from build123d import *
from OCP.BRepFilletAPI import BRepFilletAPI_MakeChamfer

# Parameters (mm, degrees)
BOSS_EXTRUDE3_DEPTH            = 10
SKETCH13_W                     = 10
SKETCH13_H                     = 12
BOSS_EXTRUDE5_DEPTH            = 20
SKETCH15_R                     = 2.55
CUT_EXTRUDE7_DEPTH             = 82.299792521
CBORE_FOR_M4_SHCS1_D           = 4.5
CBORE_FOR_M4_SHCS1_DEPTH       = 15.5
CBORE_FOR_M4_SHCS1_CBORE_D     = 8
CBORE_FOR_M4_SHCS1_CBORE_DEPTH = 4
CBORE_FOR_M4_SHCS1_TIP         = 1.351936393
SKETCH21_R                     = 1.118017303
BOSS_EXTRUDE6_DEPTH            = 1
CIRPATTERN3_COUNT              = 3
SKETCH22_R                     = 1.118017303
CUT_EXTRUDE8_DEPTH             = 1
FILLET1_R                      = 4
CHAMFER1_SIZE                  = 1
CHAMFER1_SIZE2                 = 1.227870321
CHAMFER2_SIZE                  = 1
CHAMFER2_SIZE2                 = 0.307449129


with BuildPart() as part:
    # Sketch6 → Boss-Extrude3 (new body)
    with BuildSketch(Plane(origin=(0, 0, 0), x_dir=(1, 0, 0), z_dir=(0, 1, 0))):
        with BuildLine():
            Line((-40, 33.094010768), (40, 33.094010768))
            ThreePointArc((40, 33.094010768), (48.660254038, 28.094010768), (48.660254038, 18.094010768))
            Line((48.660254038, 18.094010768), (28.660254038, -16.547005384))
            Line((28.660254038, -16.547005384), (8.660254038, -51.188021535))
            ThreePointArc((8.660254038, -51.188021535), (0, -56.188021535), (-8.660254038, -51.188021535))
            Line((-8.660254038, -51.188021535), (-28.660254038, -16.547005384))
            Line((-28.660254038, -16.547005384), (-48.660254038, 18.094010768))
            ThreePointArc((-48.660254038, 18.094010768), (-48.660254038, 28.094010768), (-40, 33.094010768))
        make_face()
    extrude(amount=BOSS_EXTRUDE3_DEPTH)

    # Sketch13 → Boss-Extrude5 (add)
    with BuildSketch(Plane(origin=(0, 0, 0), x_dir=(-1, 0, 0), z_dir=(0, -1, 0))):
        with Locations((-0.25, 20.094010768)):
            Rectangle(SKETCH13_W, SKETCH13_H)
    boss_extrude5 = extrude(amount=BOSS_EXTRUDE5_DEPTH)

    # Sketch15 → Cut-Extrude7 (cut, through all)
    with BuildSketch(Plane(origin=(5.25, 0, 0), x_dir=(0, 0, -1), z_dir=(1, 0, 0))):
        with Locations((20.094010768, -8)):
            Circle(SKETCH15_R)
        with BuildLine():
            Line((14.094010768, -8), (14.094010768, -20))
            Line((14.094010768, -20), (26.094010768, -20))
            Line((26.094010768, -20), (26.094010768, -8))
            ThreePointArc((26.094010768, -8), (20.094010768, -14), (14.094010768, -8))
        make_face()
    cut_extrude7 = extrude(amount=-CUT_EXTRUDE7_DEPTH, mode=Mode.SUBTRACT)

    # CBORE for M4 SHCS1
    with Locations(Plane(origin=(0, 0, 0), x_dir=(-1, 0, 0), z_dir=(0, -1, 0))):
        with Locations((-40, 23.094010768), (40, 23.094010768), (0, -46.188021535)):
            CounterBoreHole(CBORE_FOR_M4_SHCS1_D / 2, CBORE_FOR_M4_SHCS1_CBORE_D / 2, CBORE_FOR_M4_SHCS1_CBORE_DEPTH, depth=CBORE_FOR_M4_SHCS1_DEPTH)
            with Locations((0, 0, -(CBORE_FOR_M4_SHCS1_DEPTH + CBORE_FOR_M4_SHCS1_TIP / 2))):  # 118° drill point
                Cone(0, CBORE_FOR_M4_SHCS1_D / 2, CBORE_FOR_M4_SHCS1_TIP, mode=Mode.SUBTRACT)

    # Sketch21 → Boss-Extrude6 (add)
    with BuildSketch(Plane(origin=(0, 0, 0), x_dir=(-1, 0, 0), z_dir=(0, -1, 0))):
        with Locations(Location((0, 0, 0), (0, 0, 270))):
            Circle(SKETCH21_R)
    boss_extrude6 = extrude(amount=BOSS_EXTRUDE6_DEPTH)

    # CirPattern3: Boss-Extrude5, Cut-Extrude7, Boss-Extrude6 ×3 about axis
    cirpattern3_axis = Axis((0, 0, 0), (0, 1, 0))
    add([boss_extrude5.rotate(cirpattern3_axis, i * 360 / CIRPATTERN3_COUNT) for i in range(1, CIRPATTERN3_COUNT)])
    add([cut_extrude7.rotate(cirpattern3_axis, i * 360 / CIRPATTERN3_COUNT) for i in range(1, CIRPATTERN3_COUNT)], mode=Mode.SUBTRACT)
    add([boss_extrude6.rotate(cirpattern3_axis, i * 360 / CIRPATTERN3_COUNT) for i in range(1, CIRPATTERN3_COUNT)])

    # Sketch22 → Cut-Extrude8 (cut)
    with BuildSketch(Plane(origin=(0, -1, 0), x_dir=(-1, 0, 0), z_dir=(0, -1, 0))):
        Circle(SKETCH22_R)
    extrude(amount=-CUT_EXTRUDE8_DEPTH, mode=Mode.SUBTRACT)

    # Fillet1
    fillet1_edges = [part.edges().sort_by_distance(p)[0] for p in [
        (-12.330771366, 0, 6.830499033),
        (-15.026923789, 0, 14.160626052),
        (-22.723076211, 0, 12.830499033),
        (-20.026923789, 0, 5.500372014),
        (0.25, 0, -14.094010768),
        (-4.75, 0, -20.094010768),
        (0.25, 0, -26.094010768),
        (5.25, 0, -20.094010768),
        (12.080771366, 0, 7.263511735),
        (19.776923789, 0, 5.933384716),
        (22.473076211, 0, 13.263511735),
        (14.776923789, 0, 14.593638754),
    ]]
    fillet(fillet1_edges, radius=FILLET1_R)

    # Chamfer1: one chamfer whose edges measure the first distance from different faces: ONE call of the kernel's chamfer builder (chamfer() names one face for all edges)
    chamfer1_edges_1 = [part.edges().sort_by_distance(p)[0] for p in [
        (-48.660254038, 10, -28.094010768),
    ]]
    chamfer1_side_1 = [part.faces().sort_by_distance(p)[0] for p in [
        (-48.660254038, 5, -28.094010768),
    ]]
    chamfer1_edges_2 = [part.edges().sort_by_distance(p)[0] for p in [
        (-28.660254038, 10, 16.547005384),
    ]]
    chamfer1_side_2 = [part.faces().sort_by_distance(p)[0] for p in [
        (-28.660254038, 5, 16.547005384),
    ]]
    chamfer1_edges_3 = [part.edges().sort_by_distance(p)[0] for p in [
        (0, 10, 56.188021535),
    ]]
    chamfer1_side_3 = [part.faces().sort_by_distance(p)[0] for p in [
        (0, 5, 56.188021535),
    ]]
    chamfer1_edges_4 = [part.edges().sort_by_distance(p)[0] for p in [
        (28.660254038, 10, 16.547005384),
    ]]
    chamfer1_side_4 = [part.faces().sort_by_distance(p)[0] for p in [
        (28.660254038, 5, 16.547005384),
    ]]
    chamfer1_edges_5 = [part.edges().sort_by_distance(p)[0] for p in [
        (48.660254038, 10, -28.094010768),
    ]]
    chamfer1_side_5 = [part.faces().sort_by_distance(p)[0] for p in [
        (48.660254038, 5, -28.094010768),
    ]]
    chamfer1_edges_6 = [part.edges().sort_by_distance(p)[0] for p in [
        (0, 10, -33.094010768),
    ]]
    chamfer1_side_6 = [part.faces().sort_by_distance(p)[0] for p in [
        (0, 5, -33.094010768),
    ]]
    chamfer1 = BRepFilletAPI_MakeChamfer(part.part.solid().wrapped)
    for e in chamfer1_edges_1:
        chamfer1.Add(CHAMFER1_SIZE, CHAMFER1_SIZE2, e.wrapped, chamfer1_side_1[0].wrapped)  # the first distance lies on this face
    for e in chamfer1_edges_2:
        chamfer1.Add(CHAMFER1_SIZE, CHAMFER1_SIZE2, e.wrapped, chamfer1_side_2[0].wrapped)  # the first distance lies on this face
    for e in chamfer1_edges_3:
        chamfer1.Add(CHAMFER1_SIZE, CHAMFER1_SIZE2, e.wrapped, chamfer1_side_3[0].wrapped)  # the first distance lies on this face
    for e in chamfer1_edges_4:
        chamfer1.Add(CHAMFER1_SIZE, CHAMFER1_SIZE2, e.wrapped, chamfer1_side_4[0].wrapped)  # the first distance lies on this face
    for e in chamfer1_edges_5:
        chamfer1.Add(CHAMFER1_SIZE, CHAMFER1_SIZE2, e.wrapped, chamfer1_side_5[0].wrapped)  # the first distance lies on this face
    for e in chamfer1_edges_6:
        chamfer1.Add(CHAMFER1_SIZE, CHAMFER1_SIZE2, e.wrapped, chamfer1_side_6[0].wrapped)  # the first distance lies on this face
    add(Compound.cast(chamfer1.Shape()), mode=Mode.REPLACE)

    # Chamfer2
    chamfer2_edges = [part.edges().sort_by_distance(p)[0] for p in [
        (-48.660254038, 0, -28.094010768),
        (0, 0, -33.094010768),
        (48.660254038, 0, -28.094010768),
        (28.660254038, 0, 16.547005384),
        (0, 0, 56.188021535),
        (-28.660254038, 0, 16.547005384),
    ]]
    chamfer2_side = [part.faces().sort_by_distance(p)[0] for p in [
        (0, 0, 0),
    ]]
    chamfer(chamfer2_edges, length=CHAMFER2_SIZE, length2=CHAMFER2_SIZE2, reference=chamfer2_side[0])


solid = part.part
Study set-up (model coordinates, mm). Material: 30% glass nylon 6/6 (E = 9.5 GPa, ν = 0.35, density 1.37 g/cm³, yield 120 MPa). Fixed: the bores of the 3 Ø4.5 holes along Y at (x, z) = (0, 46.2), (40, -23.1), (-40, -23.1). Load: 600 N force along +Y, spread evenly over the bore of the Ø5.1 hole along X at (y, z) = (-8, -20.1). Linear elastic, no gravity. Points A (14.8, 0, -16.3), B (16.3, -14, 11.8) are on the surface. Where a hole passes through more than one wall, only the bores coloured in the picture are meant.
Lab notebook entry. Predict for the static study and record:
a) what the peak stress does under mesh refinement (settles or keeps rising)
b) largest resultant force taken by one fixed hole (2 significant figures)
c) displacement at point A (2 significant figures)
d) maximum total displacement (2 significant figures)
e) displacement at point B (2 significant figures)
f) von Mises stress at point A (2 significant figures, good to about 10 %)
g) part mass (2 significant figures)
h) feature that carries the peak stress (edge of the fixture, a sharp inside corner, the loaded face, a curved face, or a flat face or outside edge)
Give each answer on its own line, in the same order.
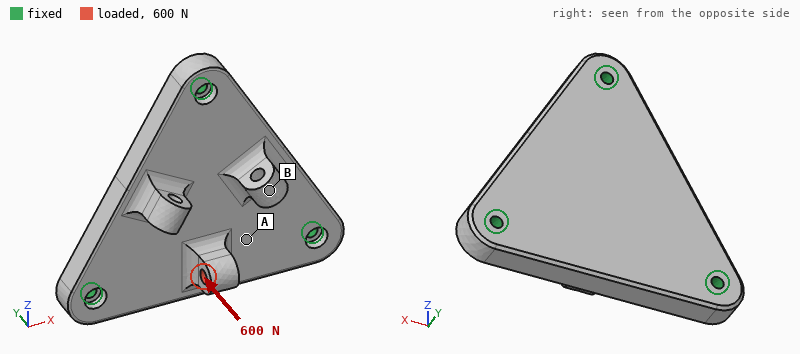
keeps rising
380 N
0.063 mm
0.11 mm
0.037 mm
6.2 MPa
80 g
edge of the fixture
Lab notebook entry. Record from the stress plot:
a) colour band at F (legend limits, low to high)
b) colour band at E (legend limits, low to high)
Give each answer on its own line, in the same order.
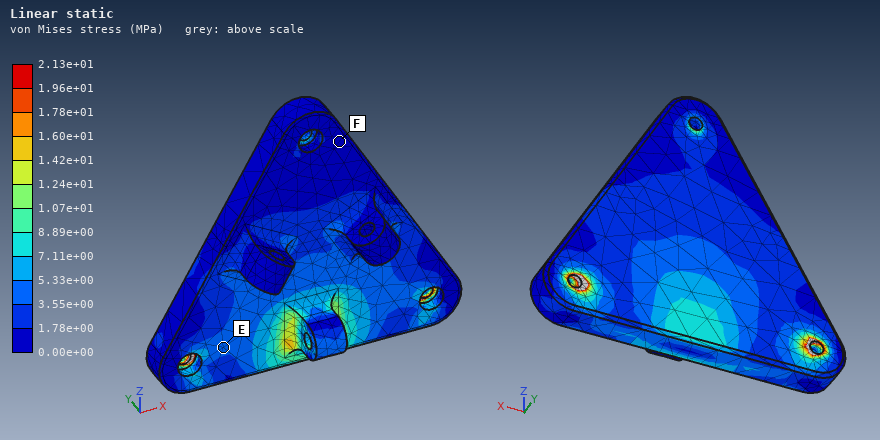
0.00e+00 to 1.78e+00 MPa
3.55e+00 to 5.33e+00 MPa
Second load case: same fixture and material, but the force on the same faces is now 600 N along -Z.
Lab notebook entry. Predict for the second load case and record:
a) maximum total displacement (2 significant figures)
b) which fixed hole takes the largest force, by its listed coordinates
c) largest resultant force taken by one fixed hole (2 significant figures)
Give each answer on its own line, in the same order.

0.10 mm
(0, 46.2)
380 N
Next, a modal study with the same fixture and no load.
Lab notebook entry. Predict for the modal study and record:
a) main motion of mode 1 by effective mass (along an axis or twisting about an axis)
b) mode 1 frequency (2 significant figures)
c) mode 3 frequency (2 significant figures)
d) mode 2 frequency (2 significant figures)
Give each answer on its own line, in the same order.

along Y
2500 Hz
3700 Hz
3700 Hz
